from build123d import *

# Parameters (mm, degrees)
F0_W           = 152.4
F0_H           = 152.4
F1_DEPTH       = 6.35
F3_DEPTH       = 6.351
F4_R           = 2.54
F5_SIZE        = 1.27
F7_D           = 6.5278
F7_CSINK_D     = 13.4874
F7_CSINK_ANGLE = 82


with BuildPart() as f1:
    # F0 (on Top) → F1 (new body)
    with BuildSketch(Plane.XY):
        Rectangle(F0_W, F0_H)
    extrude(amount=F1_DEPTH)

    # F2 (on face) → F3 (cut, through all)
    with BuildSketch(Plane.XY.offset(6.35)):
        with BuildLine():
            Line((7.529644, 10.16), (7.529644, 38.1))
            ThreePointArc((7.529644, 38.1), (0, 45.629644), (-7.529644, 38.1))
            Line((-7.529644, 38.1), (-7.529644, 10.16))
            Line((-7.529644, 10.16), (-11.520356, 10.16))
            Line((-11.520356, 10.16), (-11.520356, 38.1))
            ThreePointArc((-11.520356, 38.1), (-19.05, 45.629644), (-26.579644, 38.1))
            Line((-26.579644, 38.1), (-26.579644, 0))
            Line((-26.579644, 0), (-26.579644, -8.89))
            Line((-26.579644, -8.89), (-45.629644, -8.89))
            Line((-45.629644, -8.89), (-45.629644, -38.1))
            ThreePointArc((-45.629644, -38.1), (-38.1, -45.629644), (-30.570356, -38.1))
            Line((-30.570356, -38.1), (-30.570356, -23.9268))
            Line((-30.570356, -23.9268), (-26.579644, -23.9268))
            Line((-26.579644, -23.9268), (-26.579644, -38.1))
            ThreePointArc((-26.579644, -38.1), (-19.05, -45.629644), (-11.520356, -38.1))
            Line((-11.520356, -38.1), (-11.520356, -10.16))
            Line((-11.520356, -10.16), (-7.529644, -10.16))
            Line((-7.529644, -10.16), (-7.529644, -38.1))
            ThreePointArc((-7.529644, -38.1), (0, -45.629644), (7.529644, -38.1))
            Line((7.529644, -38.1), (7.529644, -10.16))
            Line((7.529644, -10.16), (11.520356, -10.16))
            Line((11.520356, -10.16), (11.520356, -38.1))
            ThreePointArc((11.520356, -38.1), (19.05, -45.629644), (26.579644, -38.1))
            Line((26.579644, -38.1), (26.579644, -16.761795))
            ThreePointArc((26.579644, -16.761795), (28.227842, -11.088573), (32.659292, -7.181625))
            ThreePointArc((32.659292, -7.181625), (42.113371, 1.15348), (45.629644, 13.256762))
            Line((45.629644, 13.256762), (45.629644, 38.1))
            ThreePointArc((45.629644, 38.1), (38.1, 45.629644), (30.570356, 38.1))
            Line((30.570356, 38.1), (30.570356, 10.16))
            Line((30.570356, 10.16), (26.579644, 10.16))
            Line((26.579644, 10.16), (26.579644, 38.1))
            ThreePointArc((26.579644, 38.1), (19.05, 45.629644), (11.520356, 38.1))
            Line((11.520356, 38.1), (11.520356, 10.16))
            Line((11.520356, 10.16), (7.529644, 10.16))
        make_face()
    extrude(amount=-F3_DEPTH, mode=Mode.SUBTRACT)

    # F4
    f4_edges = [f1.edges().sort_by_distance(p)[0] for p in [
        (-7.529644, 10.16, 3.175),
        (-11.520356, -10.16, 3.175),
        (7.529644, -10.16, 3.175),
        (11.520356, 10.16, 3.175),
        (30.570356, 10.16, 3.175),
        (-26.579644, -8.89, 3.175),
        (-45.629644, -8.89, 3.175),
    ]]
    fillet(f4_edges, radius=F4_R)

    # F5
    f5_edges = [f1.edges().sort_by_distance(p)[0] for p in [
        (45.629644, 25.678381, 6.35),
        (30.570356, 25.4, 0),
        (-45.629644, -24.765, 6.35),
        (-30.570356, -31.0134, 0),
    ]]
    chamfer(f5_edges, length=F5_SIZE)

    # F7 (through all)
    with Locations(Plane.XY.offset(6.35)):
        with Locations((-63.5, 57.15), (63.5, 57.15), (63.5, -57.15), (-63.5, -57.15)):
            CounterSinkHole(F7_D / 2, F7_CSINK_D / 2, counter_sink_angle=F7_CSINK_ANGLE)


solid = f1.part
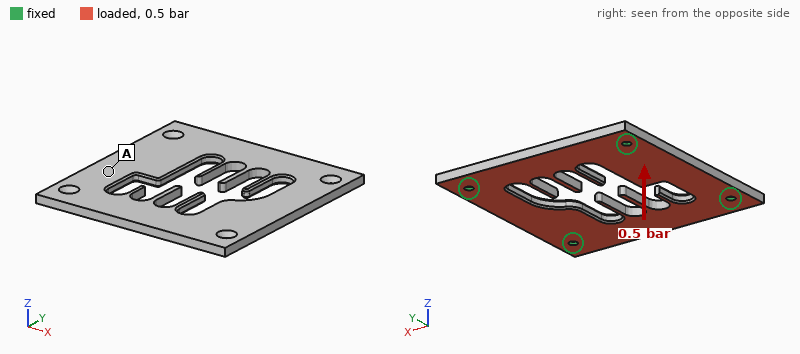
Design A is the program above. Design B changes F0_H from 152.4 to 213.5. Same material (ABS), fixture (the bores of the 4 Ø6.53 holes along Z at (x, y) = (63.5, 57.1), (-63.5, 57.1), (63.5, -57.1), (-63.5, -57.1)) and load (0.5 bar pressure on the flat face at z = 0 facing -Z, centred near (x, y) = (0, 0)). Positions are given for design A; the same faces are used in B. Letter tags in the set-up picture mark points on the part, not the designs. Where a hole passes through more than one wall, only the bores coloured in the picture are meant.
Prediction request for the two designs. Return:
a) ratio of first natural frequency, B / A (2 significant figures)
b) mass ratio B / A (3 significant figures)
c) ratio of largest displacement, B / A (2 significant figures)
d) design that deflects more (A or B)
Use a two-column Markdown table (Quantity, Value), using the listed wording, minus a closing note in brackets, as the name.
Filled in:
| Quantity | Value |
|---|---|
| ratio of first natural frequency, B / A | 0.72 |
| mass ratio B / A | 1.54 |
| ratio of largest displacement, B / A | 1.3 |
| design that deflects more | B |
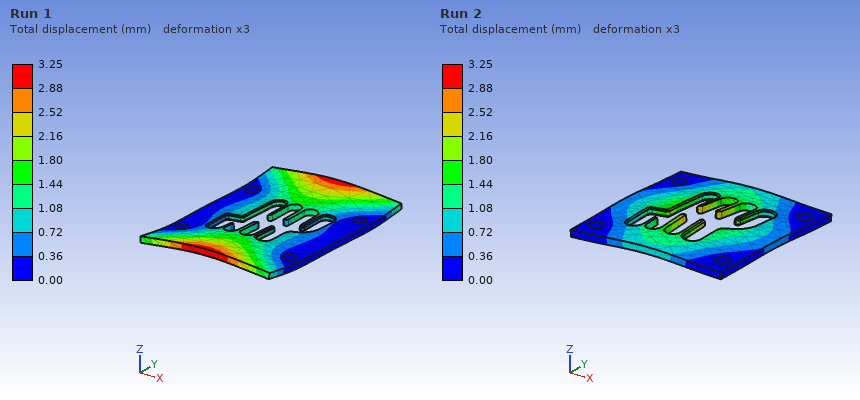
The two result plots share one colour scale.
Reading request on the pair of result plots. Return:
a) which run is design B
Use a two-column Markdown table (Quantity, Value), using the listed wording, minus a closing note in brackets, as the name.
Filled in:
| Quantity | Value |
|---|---|
| which run is design B | Run 1 |
